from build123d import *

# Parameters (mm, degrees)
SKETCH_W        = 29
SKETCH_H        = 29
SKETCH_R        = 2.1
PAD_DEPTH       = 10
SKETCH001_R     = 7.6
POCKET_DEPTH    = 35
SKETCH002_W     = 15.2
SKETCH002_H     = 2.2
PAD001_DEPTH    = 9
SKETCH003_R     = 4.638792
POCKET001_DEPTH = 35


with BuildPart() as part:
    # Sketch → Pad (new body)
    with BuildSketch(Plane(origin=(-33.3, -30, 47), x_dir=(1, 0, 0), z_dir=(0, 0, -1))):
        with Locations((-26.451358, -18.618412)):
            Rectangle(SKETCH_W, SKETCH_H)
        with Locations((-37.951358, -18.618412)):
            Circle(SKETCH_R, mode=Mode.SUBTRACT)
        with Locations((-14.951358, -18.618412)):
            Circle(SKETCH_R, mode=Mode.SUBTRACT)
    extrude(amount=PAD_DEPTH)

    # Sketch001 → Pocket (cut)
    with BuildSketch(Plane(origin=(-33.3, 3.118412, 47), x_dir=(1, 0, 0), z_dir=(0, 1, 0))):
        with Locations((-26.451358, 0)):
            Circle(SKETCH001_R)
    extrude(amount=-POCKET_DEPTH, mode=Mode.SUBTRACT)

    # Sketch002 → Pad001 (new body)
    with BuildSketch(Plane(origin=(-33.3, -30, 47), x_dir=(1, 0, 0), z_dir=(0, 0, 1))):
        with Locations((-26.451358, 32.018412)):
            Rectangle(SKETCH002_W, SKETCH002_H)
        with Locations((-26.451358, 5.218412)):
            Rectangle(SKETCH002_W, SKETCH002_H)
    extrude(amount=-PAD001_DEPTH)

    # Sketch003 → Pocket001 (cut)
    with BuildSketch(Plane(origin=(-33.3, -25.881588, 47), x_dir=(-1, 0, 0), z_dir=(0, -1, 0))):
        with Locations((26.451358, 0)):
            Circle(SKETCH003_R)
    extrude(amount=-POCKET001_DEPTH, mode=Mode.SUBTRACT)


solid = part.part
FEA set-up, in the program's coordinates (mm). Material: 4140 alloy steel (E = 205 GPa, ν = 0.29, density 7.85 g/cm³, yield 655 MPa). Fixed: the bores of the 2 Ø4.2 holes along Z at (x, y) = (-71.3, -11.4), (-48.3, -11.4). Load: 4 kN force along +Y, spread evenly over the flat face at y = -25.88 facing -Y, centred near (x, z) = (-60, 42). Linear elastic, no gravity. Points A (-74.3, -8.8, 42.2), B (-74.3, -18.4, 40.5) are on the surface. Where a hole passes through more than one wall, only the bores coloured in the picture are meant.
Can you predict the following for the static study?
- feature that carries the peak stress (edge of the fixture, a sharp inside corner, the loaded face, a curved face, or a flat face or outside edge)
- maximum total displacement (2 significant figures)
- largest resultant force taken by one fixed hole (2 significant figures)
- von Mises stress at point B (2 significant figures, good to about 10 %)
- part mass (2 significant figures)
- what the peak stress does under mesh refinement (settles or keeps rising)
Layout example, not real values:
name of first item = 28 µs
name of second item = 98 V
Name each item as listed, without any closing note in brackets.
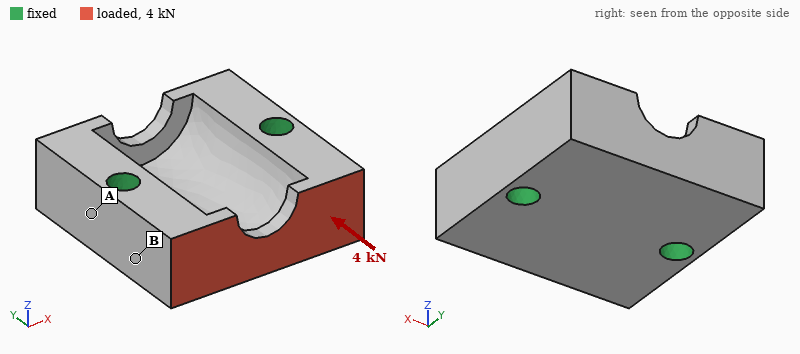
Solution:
feature that carries the peak stress = a sharp inside corner
maximum total displacement = 5.1 µm
largest resultant force taken by one fixed hole = 2.0 kN
von Mises stress at point B = 14 MPa
part mass = 45 g
what the peak stress does under mesh refinement = keeps rising
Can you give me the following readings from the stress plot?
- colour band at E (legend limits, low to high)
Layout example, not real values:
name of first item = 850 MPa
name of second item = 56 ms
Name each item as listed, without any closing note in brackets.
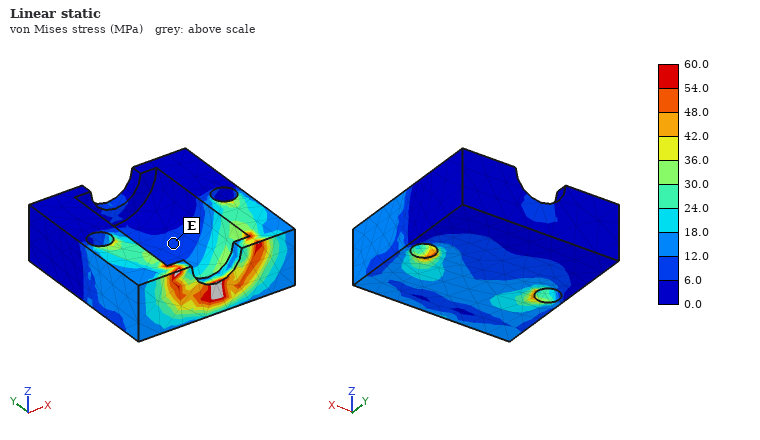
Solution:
colour band at E = 6.0 to 12.0 MPa
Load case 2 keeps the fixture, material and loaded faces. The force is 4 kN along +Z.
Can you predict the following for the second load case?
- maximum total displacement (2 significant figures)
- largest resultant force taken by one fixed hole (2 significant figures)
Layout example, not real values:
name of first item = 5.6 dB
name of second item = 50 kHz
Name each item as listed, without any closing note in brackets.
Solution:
maximum total displacement = 22 µm
largest resultant force taken by one fixed hole = 2.0 kN
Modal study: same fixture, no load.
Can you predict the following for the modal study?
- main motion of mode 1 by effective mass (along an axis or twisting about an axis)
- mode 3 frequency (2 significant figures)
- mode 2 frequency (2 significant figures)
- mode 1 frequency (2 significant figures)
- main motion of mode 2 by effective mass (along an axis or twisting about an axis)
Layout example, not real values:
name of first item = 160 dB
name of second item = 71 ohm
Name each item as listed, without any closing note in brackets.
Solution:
main motion of mode 1 by effective mass = twisting about X
mode 3 frequency = 32 kHz
mode 2 frequency = 30 kHz
mode 1 frequency = 27 kHz
main motion of mode 2 by effective mass = along Z
